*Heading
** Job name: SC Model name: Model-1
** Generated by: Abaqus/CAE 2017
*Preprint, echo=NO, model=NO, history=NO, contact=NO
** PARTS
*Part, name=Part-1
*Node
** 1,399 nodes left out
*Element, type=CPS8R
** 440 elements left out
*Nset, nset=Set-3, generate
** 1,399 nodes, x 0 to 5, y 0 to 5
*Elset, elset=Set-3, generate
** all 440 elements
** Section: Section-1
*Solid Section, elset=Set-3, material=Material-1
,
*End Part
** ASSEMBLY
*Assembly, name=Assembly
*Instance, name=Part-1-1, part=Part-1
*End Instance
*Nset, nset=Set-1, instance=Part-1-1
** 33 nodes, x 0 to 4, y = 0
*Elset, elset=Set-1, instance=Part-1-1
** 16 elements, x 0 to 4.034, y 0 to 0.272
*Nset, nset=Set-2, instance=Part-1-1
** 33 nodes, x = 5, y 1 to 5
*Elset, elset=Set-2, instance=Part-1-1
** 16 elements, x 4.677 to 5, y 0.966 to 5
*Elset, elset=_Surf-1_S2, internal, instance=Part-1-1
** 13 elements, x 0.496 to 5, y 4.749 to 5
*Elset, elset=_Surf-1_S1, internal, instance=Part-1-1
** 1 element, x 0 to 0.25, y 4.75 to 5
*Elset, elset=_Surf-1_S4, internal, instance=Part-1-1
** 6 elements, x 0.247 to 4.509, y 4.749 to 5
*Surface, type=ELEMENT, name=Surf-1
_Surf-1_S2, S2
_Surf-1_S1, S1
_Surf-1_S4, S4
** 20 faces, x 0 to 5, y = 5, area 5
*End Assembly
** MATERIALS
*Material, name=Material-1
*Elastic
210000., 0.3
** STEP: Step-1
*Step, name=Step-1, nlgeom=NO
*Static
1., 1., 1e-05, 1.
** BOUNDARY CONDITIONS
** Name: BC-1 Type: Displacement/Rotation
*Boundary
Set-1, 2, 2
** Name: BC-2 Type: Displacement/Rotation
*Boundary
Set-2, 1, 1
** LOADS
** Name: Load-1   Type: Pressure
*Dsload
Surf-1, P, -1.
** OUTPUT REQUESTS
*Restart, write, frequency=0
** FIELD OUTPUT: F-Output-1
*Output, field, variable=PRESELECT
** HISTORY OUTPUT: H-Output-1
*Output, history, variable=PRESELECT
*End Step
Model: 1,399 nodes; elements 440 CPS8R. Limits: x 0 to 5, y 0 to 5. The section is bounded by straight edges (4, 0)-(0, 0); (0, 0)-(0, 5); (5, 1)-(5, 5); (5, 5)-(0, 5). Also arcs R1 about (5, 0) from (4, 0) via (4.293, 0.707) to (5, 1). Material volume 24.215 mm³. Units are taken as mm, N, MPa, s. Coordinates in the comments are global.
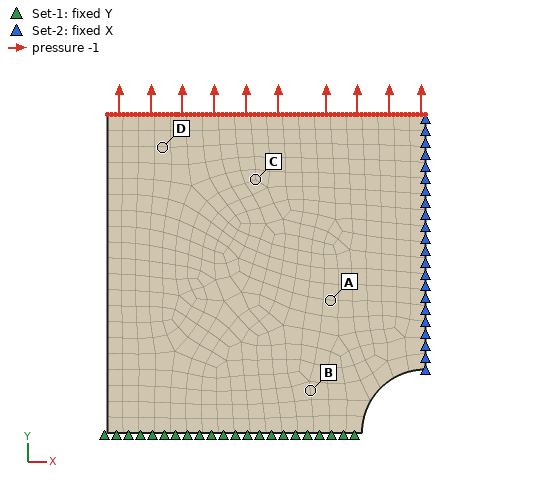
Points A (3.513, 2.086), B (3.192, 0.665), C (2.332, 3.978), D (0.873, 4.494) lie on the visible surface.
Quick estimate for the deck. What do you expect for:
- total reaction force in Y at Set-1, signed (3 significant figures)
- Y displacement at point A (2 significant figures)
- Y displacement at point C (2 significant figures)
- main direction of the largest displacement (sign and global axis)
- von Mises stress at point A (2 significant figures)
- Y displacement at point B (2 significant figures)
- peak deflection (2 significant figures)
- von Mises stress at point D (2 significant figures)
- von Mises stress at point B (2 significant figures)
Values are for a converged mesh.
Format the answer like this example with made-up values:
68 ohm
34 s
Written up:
-5.00 N
1.4e-05 mm
2.1e-05 mm
+Y
1.2 MPa
4.2e-06 mm
2.9e-05 mm
1.0 MPa
1.3 MPa
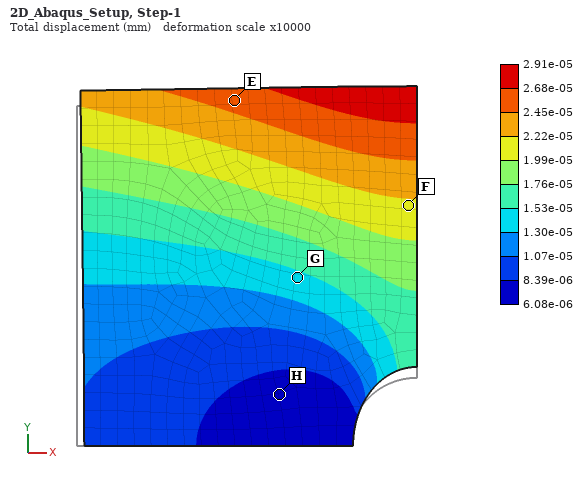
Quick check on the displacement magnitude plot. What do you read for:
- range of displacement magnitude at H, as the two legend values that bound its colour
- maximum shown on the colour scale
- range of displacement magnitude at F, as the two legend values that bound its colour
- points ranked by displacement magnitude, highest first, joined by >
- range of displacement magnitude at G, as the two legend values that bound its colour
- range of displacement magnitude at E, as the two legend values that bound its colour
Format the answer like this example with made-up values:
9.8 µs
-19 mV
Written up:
6.08e-06 to 8.39e-06 mm
2.91e-05 mm
1.99e-05 to 2.22e-05 mm
E > F > G > H
1.30e-05 to 1.53e-05 mm
2.45e-05 to 2.68e-05 mm
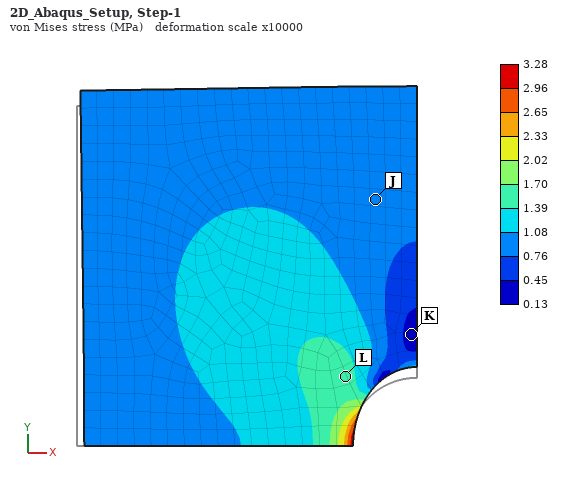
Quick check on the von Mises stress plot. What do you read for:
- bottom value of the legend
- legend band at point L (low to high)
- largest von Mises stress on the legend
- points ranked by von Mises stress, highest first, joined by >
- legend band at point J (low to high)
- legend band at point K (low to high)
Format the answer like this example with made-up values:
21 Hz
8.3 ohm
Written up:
0.13 MPa
1.39 to 1.70 MPa
3.28 MPa
L > J > K
0.76 to 1.08 MPa
0.13 to 0.45 MPa
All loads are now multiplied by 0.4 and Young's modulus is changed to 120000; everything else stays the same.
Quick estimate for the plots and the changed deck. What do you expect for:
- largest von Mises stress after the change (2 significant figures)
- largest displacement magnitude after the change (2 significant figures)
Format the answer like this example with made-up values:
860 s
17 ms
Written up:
1.3 MPa
2.0e-05 mm
